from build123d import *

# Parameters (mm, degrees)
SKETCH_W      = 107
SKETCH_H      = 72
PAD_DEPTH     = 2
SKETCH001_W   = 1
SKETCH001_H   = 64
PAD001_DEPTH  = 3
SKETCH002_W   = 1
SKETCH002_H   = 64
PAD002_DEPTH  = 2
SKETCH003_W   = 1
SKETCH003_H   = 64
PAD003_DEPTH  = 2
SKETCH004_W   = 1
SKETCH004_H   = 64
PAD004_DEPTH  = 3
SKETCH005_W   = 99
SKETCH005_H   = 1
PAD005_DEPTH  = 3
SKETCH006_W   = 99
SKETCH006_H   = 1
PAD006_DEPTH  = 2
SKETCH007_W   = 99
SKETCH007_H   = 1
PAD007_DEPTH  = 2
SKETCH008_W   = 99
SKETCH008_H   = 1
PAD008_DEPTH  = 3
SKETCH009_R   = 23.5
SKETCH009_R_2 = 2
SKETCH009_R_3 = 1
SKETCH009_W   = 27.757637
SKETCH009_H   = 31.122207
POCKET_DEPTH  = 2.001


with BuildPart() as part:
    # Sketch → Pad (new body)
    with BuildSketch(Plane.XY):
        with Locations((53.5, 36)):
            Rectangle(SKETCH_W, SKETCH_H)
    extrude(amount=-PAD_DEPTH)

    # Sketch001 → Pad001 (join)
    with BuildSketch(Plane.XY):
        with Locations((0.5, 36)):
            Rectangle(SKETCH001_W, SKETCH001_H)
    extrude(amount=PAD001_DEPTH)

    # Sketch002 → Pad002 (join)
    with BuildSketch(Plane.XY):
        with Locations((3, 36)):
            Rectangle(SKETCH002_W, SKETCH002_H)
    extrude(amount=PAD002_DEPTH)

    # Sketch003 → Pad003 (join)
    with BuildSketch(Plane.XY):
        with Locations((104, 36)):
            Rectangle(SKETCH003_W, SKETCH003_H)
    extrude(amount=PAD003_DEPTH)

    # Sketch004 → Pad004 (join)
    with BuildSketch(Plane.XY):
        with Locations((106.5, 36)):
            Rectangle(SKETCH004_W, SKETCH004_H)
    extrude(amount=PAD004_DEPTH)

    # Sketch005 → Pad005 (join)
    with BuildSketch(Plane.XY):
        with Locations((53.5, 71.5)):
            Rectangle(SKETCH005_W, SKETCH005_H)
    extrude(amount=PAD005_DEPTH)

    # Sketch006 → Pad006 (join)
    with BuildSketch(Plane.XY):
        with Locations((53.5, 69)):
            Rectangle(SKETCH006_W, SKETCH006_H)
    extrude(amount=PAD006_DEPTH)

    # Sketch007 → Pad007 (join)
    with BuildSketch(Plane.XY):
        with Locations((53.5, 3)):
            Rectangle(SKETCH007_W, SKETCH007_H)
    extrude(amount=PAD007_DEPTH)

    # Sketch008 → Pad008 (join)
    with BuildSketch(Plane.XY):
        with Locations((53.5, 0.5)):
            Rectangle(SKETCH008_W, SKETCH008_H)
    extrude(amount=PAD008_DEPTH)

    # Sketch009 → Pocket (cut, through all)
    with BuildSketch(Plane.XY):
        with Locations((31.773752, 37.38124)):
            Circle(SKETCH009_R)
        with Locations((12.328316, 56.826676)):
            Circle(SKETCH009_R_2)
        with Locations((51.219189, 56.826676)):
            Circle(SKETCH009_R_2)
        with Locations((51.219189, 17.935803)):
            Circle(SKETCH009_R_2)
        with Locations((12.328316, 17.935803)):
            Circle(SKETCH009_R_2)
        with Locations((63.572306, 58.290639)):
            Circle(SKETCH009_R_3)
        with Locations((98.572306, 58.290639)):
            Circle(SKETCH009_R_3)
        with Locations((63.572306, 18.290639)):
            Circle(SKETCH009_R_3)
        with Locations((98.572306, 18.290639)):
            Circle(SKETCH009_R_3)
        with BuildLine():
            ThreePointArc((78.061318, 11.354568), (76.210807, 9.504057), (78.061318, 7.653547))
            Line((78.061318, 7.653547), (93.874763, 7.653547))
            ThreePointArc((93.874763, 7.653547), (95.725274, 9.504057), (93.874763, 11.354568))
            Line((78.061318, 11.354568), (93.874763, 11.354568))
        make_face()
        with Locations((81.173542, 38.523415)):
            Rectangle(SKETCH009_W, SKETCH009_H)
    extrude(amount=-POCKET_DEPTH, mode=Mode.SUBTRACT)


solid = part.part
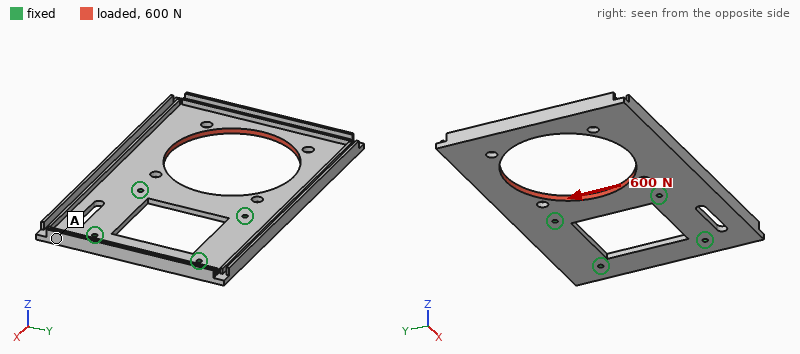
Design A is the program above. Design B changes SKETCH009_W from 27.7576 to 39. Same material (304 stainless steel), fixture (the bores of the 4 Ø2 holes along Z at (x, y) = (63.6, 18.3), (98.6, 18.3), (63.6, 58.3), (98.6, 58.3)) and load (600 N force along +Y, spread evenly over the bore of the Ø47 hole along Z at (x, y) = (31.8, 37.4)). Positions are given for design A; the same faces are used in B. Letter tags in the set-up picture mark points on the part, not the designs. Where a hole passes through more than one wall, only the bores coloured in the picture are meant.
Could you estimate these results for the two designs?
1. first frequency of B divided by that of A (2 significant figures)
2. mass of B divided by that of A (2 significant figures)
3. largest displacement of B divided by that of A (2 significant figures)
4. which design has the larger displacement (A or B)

0.99
0.94
1.1
B
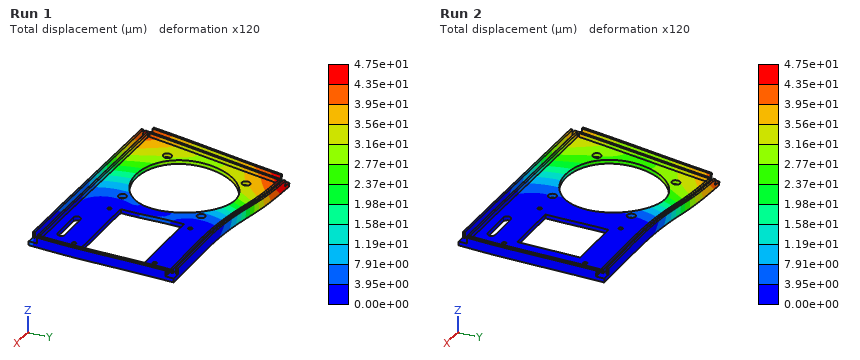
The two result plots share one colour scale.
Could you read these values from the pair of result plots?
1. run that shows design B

Run 1
